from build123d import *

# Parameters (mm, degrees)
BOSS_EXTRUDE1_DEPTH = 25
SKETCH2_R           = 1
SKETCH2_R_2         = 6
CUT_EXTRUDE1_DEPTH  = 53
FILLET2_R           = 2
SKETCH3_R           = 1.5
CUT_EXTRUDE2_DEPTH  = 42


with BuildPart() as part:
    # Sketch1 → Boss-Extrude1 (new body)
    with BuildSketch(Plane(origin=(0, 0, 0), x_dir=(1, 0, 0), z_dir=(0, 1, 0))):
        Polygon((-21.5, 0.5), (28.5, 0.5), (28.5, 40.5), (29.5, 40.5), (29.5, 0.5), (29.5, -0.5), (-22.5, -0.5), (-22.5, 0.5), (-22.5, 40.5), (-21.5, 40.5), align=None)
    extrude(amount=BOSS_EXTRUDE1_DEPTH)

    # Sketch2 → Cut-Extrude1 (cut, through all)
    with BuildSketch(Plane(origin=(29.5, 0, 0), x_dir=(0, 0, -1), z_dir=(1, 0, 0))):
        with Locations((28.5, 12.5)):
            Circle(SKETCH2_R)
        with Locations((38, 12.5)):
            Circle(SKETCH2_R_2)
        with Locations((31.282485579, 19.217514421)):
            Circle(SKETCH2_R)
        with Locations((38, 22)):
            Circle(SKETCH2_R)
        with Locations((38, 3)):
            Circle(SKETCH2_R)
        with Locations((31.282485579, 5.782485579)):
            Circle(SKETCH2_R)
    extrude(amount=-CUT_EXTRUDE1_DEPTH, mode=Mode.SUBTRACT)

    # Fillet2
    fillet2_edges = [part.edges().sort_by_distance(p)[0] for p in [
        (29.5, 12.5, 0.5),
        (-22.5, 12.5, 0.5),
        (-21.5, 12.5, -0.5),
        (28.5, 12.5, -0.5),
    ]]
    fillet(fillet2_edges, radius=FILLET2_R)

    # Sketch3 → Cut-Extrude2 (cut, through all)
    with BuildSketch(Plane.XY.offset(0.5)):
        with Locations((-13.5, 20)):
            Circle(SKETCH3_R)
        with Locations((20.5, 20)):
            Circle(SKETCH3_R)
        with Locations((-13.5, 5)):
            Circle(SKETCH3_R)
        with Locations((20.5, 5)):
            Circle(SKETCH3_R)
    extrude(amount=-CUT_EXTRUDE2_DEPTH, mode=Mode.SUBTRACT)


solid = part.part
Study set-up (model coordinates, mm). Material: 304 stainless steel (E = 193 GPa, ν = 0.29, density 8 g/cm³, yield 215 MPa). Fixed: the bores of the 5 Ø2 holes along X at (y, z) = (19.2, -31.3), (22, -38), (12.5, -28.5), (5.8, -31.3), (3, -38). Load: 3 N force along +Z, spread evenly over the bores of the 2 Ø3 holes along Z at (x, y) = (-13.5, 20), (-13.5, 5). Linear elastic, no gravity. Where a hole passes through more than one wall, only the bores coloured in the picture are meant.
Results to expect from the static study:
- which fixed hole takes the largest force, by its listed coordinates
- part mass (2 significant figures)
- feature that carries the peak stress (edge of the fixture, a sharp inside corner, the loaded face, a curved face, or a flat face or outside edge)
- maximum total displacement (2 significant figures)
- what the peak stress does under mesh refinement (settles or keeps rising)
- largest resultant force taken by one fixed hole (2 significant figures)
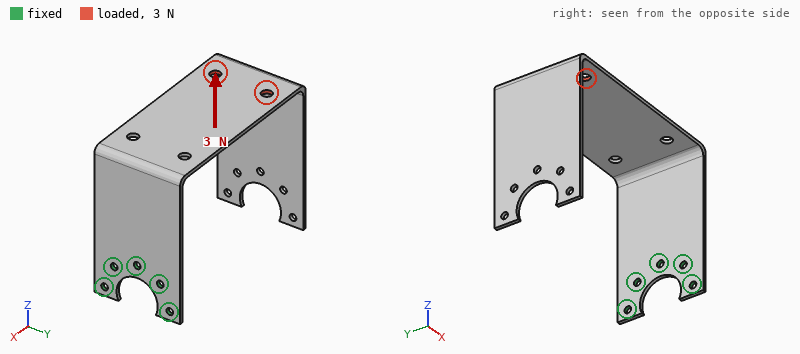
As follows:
(12.5, -28.5)
25 g
edge of the fixture
0.82 mm
keeps rising
10 N
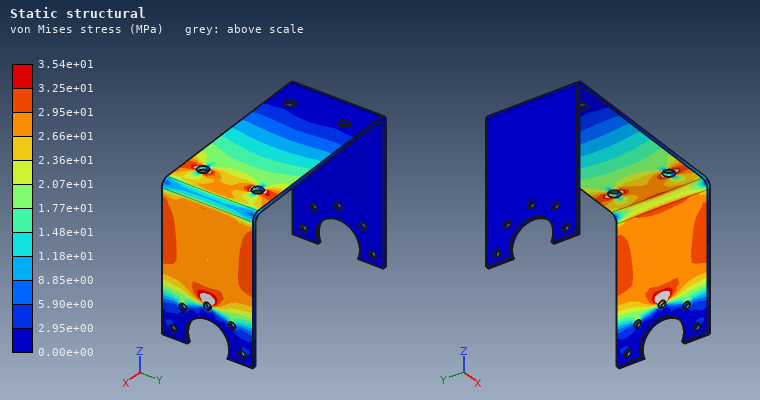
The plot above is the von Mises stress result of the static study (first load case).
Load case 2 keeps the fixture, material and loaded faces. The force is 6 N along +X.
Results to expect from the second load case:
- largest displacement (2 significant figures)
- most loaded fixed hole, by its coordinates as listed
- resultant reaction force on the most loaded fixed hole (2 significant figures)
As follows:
0.33 mm
(12.5, -28.5)
15 N
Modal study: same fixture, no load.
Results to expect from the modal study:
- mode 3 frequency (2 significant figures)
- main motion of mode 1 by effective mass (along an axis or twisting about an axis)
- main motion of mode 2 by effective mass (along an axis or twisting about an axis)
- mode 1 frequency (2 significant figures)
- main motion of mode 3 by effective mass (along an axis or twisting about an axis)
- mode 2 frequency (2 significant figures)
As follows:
260 Hz
along Z
along Y
89 Hz
along X
140 Hz
